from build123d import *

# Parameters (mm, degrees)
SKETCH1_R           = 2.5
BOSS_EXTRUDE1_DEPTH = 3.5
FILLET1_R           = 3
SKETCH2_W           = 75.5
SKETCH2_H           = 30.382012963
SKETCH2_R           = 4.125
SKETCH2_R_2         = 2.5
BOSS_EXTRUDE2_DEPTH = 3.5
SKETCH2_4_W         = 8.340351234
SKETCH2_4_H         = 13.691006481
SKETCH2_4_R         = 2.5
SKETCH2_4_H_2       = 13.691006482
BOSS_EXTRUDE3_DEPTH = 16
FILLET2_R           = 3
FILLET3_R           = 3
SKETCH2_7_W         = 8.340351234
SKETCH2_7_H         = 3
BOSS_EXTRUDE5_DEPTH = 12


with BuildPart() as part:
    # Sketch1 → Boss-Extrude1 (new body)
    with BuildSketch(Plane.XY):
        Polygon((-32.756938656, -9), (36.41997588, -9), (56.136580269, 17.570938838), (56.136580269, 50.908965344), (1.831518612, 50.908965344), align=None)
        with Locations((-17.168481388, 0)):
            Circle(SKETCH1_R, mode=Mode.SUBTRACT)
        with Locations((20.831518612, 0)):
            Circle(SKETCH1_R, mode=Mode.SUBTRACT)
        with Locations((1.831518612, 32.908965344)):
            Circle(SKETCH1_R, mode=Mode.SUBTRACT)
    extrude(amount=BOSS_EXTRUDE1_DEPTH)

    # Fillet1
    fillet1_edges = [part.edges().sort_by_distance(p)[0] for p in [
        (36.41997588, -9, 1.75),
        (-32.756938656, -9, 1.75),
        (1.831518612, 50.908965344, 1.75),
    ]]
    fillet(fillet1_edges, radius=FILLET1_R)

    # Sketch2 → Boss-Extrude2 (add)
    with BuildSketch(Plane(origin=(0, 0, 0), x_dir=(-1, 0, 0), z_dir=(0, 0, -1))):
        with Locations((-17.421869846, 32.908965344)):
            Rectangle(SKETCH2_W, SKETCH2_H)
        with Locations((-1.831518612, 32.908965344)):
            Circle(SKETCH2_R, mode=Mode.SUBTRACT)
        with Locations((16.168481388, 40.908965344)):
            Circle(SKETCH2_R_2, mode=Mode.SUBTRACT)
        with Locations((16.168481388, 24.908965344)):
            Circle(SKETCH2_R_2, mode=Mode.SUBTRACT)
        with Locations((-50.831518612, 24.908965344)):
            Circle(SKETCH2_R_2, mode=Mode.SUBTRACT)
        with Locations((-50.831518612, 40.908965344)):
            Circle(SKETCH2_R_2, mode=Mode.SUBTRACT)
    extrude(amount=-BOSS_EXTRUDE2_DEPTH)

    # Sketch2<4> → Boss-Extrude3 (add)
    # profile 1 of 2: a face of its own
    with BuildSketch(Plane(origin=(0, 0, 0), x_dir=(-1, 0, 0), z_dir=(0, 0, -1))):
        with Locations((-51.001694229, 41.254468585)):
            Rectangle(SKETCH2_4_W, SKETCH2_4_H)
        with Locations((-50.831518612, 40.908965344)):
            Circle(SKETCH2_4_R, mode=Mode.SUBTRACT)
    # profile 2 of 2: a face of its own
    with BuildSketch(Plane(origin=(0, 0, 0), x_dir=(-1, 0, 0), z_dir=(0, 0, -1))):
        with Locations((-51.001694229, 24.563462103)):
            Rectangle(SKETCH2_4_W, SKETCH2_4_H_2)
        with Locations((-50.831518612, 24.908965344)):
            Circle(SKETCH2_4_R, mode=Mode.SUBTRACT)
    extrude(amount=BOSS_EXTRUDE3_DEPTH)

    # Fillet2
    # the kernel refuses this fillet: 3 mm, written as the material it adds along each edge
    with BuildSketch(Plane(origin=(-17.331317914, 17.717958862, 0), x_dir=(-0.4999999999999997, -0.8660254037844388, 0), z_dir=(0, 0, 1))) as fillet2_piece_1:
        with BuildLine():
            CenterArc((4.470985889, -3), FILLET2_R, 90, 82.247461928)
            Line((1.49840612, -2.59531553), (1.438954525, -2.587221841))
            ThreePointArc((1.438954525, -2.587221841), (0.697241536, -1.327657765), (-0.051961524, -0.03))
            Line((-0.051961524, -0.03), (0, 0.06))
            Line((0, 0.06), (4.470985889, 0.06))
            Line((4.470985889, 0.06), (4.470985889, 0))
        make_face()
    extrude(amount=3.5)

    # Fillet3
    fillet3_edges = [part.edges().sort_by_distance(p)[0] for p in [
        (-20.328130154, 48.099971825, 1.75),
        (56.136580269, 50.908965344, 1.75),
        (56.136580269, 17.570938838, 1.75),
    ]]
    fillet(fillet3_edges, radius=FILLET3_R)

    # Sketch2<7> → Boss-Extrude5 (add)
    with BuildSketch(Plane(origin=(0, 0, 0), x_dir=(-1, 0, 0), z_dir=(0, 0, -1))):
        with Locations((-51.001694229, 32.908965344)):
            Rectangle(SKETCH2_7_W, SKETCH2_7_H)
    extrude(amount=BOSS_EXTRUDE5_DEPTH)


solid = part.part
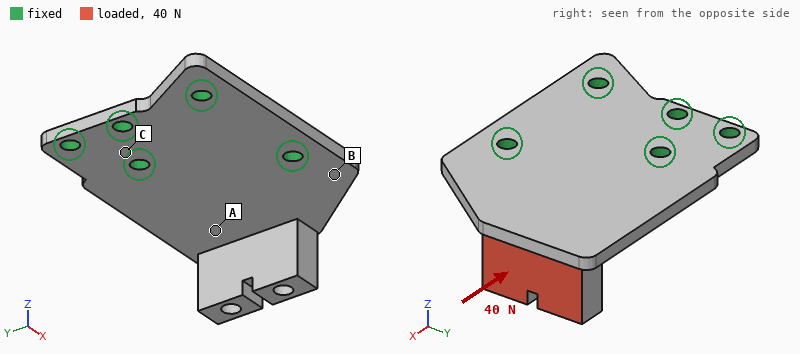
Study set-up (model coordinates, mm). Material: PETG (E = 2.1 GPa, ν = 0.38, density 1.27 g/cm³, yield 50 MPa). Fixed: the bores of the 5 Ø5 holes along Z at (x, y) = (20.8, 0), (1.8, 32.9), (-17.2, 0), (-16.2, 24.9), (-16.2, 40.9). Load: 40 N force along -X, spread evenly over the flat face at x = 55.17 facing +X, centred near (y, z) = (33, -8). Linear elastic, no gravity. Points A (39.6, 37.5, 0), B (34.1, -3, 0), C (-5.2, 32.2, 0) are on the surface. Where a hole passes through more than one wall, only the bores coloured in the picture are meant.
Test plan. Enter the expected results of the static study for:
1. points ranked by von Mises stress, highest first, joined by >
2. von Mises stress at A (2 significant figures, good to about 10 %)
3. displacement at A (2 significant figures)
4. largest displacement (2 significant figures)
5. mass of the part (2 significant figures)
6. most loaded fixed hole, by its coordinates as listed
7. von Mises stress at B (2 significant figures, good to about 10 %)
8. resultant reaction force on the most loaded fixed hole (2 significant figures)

A > B > C
3.7 MPa
0.38 mm
1.1 mm
23 g
(1.8, 32.9)
2.9 MPa
23 N
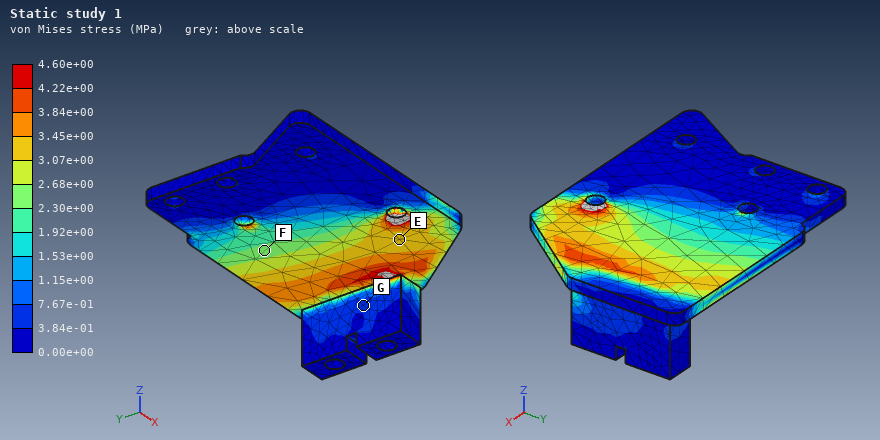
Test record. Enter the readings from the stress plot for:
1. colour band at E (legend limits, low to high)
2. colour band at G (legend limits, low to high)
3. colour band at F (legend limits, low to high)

3.07e+00 to 3.45e+00 MPa
3.84e-01 to 7.67e-01 MPa
2.30e+00 to 2.68e+00 MPa
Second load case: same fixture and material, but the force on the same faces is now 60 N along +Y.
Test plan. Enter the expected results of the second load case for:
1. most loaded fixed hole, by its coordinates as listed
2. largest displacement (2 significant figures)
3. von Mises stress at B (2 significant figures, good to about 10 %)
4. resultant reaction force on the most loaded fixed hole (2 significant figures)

(20.8, 0)
1.1 mm
1.4 MPa
75 N
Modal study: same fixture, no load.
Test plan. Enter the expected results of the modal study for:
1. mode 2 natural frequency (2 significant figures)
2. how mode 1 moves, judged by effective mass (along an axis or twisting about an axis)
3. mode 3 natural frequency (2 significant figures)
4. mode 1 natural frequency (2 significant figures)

730 Hz
along Z
1200 Hz
240 Hz
